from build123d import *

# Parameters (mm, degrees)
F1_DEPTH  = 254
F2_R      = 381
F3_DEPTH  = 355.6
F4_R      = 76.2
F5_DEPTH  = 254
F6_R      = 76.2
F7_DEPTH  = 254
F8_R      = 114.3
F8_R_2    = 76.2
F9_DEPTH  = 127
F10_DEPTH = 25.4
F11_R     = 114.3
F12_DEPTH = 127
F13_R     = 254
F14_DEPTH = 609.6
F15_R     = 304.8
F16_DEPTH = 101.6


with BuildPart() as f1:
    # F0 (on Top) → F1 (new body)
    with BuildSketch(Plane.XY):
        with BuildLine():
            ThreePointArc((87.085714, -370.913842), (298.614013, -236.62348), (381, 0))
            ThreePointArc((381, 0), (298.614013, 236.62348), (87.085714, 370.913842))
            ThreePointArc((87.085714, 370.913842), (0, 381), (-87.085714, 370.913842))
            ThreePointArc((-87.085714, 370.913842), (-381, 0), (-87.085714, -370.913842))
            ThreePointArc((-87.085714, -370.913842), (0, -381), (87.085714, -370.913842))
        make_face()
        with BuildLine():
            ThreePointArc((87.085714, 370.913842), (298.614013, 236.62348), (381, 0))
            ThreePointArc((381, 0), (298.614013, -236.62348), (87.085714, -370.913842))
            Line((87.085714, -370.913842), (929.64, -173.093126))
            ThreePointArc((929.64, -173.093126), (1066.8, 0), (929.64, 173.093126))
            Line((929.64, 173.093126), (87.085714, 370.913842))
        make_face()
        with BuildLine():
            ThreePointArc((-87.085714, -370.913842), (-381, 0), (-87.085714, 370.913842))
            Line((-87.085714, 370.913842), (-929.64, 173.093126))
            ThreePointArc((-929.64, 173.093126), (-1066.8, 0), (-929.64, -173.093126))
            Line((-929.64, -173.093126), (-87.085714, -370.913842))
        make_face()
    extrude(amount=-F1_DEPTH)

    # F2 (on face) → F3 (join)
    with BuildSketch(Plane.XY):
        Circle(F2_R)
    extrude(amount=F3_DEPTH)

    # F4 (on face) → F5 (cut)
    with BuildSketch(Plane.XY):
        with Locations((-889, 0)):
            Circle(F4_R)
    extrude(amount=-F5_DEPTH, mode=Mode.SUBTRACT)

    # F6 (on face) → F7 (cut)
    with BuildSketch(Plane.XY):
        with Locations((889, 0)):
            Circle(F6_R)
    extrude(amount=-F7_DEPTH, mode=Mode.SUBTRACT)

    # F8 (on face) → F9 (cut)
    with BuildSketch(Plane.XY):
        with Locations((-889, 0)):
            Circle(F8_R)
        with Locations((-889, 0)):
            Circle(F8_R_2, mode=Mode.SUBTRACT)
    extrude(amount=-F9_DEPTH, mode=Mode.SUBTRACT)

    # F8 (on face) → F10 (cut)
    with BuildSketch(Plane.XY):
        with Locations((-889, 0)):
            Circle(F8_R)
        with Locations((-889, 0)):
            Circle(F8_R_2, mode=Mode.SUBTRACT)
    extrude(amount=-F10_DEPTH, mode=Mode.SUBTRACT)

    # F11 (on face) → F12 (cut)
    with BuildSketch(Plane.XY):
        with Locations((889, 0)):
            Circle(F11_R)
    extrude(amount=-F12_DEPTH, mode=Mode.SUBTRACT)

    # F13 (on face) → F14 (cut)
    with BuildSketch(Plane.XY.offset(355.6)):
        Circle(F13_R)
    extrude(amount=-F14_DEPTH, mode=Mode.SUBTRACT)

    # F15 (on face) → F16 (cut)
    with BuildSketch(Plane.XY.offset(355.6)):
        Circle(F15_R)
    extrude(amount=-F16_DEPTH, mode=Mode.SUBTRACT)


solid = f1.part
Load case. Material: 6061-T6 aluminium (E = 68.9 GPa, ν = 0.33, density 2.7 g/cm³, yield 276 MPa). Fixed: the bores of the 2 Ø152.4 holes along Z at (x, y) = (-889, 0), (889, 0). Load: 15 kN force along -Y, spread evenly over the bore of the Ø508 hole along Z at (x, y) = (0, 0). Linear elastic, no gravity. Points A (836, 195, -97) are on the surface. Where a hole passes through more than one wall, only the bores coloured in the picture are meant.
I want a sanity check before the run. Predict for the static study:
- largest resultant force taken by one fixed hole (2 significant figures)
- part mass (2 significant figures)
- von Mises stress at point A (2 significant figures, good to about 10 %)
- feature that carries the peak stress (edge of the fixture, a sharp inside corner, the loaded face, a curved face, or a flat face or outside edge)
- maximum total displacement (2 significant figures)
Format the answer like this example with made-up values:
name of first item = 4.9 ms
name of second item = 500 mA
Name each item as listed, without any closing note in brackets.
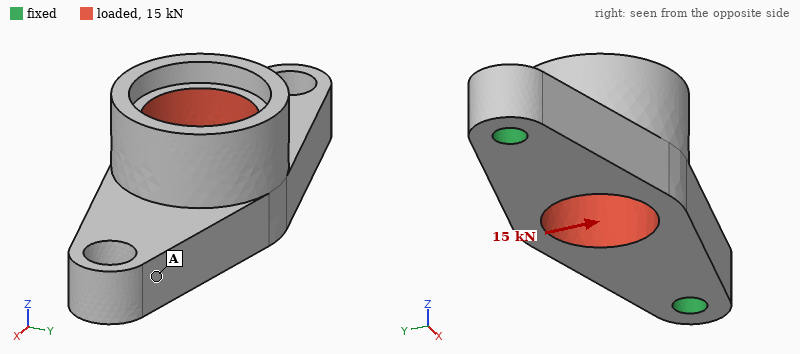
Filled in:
largest resultant force taken by one fixed hole = 7.5 kN
part mass = 810 kg
von Mises stress at point A = 0.25 MPa
feature that carries the peak stress = edge of the fixture
maximum total displacement = 18 µm
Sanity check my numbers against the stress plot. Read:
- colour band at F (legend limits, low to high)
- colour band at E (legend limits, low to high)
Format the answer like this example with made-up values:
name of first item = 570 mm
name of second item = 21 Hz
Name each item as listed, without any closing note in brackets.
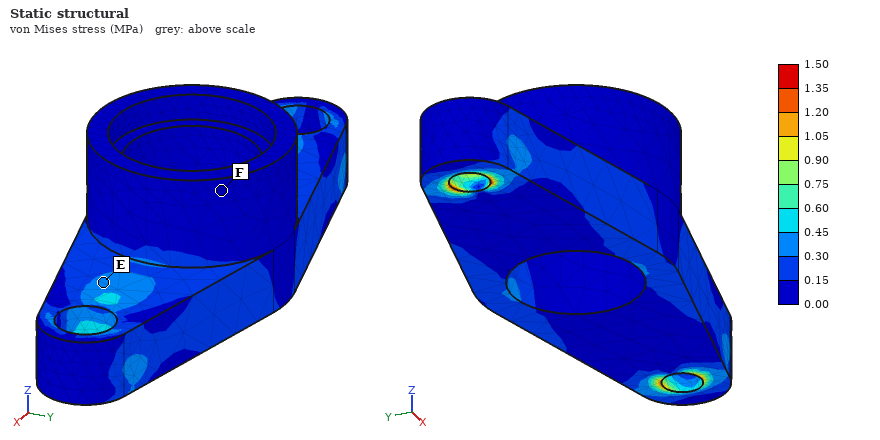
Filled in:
colour band at F = 0.00 to 0.15 MPa
colour band at E = 0.30 to 0.45 MPa
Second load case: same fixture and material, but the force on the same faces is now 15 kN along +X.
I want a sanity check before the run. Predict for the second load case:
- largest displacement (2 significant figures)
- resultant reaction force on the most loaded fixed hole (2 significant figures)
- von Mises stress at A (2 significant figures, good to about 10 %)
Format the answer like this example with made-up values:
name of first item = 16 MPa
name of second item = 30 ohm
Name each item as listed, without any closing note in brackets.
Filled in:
largest displacement = 1.5 µm
resultant reaction force on the most loaded fixed hole = 7.7 kN
von Mises stress at A = 0.037 MPa
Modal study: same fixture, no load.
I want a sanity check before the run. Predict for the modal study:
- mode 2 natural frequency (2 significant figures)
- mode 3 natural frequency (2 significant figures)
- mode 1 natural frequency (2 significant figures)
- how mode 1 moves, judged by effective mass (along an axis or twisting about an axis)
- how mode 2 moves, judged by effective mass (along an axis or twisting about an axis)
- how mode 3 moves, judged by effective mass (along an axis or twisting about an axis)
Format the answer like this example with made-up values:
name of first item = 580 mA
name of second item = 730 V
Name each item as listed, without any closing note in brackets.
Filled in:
mode 2 natural frequency = 270 Hz
mode 3 natural frequency = 490 Hz
mode 1 natural frequency = 210 Hz
how mode 1 moves, judged by effective mass = along Y
how mode 2 moves, judged by effective mass = along Z
how mode 3 moves, judged by effective mass = along Y
